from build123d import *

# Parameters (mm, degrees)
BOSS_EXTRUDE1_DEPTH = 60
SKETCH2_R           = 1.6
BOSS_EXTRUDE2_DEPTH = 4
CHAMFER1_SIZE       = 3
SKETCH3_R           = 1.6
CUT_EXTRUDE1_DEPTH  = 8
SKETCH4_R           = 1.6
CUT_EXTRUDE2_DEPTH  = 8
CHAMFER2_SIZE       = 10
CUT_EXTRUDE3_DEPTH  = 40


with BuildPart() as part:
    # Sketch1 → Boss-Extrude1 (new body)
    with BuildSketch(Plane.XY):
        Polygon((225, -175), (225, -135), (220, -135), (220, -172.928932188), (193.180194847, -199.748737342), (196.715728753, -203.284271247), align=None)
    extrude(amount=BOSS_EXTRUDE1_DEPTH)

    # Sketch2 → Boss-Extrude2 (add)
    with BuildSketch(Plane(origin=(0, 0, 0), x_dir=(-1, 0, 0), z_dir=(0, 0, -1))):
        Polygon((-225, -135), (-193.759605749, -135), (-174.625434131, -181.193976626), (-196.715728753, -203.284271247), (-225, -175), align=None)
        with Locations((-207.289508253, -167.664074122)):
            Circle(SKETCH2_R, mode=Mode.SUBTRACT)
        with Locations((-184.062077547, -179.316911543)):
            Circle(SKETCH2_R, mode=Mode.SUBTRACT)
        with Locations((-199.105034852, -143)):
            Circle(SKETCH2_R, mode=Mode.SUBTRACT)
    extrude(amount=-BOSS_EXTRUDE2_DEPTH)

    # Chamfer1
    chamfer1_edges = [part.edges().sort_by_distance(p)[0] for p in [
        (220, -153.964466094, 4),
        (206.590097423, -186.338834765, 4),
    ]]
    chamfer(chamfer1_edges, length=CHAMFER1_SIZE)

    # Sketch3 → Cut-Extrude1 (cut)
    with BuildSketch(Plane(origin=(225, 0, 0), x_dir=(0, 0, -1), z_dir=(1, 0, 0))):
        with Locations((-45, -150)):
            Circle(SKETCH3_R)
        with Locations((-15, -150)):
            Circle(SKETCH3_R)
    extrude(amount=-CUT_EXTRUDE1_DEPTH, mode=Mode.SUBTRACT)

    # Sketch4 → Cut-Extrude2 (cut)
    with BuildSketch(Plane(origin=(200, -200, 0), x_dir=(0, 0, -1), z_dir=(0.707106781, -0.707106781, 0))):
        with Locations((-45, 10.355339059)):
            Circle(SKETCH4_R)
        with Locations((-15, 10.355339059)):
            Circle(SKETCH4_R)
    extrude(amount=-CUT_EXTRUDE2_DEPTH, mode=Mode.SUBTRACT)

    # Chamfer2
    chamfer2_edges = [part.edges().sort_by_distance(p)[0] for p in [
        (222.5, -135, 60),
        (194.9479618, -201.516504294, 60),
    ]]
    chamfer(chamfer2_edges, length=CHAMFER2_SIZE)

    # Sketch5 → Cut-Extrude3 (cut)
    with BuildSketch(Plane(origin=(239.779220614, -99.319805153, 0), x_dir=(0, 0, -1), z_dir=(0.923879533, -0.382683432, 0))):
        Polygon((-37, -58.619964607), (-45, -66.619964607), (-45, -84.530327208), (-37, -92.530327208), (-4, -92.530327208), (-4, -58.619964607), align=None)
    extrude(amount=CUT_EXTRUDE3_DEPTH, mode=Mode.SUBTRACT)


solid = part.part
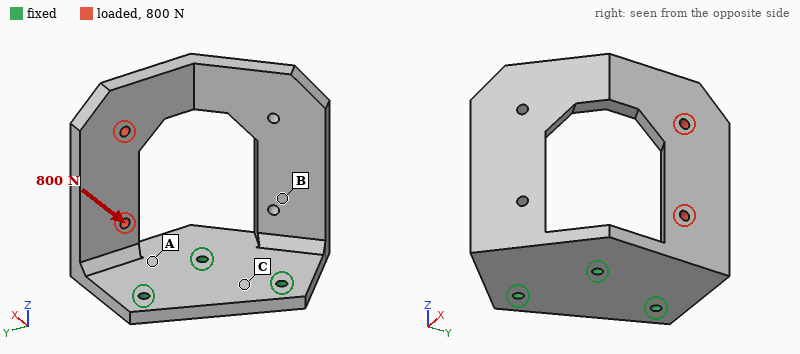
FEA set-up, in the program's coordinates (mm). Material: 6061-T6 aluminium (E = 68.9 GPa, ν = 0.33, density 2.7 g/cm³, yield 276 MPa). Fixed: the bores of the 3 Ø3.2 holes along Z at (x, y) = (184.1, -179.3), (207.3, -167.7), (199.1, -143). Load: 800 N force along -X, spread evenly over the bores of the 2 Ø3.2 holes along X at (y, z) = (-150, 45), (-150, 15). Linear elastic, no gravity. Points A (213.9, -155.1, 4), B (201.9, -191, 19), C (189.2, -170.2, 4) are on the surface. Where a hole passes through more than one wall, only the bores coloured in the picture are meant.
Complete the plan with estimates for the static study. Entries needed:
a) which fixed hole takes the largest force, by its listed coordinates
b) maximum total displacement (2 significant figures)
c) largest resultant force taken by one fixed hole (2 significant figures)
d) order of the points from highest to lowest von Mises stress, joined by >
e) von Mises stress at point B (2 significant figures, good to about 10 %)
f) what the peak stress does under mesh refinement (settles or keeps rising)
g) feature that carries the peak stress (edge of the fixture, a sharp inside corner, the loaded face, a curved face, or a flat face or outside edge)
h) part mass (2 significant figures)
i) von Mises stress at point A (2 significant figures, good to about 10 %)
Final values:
(207.3, -167.7)
0.99 mm
1.0 kN
A > B > C
51 MPa
keeps rising
edge of the fixture
63 g
99 MPa
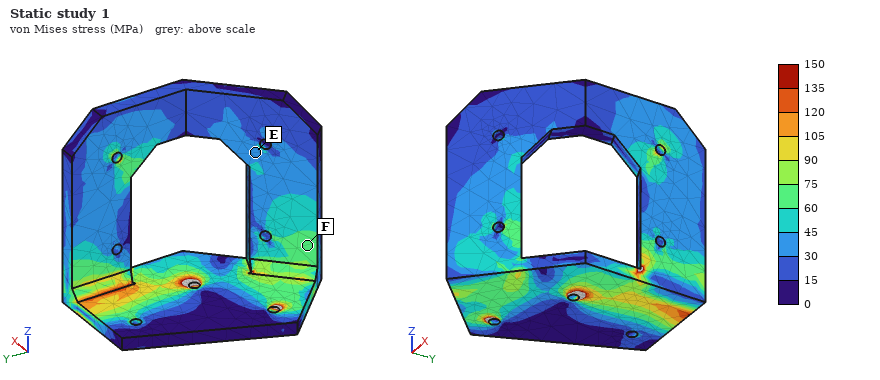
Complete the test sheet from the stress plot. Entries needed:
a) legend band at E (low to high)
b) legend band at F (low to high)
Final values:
30 to 45 MPa
60 to 75 MPa
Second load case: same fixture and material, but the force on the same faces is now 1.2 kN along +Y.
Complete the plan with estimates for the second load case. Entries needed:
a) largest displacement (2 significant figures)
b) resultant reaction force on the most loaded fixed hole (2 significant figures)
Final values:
0.69 mm
1.2 kN
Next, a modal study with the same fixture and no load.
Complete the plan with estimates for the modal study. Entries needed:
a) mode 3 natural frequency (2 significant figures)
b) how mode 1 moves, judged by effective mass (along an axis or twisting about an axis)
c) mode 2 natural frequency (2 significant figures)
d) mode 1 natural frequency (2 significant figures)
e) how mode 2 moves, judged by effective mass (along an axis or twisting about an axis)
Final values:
2400 Hz
along X
1100 Hz
890 Hz
along Y
